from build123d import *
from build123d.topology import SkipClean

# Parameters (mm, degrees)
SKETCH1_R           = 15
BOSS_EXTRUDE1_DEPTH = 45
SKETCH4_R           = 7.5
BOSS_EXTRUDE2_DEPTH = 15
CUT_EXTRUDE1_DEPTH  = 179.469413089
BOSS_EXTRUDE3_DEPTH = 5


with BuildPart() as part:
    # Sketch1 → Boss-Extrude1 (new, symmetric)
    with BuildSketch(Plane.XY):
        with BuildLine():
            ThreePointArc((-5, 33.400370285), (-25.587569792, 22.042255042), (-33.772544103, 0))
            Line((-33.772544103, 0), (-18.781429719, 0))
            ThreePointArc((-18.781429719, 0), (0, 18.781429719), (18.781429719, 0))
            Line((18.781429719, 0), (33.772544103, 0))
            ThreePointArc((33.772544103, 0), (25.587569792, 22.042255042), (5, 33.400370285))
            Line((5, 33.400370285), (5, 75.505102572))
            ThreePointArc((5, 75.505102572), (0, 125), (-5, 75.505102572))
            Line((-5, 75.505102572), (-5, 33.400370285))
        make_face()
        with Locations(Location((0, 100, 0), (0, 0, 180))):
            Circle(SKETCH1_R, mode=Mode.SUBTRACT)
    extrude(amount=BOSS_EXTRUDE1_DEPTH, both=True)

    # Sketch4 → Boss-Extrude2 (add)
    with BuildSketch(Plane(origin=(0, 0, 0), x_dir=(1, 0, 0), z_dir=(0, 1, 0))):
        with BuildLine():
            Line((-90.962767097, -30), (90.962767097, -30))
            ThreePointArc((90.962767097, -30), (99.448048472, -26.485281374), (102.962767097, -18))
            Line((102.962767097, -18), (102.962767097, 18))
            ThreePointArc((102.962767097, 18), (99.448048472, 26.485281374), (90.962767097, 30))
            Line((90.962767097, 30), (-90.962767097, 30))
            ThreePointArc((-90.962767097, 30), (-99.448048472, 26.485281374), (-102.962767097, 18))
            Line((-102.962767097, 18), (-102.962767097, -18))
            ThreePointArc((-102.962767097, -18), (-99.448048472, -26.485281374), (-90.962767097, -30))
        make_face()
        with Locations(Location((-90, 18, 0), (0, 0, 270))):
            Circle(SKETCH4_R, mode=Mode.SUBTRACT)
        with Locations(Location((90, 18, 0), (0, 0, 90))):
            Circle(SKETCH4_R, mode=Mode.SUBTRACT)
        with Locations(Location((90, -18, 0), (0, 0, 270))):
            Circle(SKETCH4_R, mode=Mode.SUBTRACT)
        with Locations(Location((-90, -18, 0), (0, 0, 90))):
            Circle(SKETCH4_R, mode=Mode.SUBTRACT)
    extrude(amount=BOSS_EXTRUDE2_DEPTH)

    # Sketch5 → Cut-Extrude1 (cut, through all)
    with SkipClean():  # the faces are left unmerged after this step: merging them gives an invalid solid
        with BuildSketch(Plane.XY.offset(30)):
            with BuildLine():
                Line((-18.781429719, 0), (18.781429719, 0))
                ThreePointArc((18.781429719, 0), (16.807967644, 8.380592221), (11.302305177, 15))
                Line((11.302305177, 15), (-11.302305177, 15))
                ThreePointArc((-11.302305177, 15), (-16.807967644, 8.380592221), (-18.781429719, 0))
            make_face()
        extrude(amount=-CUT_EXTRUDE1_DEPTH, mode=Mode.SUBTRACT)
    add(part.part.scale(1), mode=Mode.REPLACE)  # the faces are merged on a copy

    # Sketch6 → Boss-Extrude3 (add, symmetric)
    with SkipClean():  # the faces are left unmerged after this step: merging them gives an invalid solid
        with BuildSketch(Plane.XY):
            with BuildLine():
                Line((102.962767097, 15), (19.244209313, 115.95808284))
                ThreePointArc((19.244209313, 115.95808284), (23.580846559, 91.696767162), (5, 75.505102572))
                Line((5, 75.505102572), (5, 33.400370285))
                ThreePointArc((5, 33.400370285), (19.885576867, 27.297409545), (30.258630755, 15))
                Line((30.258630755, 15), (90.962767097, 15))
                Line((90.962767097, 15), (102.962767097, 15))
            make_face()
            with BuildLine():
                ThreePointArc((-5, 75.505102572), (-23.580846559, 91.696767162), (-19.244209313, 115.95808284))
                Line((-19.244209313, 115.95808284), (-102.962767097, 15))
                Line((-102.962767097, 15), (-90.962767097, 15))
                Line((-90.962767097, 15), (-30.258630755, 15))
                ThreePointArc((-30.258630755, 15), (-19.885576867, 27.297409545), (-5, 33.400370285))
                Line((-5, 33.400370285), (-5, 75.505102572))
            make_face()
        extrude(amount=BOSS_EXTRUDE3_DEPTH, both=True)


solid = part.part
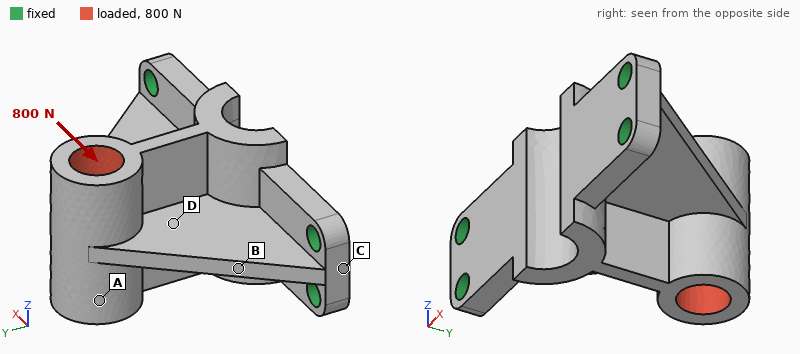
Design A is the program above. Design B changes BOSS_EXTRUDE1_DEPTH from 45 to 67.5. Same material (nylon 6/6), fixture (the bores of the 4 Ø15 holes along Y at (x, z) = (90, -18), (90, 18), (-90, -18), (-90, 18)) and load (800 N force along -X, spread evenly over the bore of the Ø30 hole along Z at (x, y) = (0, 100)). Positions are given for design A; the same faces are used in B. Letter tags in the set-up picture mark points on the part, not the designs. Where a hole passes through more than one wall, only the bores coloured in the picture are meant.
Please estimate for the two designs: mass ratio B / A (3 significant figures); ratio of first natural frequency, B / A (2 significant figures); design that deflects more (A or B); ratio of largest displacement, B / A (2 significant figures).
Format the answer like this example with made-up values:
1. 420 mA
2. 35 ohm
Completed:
1. 1.28
2. 0.79
3. B
4. 1.1
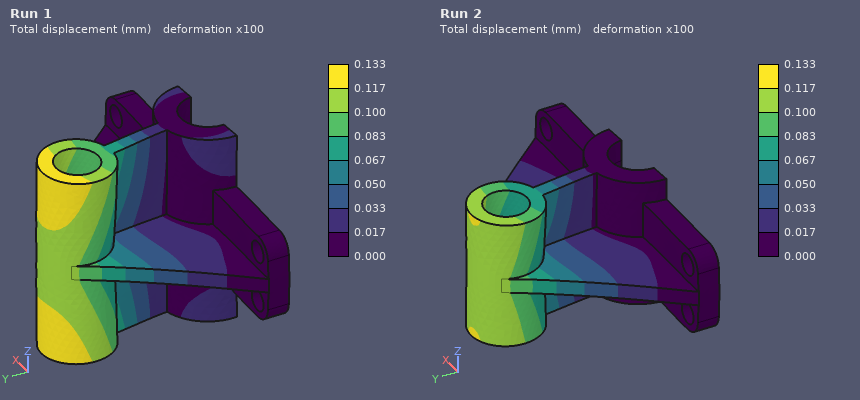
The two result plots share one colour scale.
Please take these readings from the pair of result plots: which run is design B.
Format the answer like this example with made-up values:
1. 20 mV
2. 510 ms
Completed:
1. Run 1
